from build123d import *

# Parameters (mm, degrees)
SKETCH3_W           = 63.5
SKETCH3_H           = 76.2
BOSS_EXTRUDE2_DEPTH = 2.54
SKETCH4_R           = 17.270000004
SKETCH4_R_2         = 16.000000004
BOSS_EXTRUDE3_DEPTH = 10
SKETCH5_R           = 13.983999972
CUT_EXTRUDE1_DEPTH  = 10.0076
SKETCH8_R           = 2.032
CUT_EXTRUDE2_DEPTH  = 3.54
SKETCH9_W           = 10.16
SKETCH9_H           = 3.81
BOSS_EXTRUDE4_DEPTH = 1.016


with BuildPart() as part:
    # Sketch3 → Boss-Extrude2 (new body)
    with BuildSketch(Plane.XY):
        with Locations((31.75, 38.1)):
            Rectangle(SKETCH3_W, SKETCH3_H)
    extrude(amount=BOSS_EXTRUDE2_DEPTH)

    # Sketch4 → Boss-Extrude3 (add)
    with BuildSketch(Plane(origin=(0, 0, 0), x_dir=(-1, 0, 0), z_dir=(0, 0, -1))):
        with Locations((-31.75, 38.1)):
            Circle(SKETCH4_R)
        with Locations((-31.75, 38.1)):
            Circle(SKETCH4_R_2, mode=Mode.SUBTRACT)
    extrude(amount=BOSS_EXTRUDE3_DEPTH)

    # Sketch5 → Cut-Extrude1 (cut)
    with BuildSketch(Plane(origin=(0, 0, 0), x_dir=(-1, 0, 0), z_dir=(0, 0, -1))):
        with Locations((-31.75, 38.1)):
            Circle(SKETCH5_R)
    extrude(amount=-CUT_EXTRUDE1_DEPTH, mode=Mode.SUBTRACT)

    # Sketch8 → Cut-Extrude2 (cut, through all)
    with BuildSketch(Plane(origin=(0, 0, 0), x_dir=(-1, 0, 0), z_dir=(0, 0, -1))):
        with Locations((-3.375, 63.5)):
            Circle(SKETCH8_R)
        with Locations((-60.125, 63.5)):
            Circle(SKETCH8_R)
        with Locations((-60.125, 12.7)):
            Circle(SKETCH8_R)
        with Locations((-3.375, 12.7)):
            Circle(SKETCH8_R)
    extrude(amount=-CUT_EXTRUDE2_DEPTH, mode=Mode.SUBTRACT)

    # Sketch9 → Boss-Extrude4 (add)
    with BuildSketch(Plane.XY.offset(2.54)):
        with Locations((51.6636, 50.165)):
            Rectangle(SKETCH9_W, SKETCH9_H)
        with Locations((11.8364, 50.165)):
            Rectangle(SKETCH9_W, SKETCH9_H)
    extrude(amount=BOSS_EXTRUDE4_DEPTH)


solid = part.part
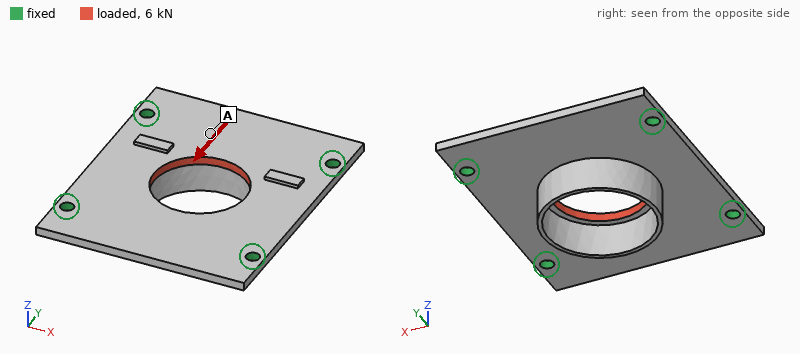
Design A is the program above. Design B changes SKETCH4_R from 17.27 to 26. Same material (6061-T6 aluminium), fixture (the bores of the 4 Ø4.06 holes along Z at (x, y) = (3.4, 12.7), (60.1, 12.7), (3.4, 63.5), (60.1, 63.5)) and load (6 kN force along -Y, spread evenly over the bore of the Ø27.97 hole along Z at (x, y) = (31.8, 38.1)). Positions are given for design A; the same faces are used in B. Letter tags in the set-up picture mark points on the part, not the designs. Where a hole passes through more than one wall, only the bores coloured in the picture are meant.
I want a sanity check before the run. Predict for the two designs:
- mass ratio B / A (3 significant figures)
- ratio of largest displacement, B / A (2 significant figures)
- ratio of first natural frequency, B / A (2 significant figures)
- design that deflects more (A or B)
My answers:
1.99
0.85
1.1
A
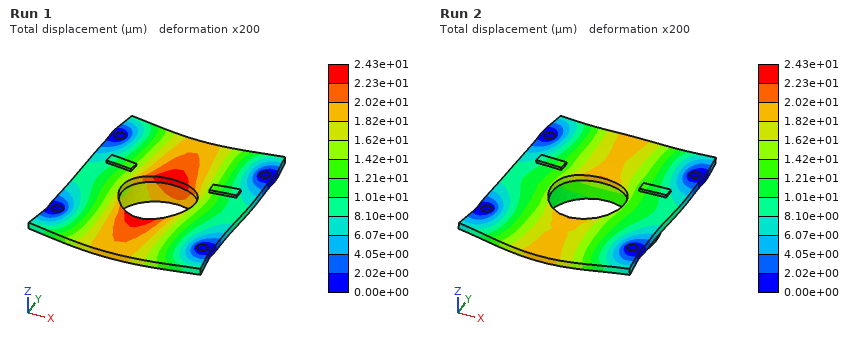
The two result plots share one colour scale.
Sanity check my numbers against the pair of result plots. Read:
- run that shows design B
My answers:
Run 2
